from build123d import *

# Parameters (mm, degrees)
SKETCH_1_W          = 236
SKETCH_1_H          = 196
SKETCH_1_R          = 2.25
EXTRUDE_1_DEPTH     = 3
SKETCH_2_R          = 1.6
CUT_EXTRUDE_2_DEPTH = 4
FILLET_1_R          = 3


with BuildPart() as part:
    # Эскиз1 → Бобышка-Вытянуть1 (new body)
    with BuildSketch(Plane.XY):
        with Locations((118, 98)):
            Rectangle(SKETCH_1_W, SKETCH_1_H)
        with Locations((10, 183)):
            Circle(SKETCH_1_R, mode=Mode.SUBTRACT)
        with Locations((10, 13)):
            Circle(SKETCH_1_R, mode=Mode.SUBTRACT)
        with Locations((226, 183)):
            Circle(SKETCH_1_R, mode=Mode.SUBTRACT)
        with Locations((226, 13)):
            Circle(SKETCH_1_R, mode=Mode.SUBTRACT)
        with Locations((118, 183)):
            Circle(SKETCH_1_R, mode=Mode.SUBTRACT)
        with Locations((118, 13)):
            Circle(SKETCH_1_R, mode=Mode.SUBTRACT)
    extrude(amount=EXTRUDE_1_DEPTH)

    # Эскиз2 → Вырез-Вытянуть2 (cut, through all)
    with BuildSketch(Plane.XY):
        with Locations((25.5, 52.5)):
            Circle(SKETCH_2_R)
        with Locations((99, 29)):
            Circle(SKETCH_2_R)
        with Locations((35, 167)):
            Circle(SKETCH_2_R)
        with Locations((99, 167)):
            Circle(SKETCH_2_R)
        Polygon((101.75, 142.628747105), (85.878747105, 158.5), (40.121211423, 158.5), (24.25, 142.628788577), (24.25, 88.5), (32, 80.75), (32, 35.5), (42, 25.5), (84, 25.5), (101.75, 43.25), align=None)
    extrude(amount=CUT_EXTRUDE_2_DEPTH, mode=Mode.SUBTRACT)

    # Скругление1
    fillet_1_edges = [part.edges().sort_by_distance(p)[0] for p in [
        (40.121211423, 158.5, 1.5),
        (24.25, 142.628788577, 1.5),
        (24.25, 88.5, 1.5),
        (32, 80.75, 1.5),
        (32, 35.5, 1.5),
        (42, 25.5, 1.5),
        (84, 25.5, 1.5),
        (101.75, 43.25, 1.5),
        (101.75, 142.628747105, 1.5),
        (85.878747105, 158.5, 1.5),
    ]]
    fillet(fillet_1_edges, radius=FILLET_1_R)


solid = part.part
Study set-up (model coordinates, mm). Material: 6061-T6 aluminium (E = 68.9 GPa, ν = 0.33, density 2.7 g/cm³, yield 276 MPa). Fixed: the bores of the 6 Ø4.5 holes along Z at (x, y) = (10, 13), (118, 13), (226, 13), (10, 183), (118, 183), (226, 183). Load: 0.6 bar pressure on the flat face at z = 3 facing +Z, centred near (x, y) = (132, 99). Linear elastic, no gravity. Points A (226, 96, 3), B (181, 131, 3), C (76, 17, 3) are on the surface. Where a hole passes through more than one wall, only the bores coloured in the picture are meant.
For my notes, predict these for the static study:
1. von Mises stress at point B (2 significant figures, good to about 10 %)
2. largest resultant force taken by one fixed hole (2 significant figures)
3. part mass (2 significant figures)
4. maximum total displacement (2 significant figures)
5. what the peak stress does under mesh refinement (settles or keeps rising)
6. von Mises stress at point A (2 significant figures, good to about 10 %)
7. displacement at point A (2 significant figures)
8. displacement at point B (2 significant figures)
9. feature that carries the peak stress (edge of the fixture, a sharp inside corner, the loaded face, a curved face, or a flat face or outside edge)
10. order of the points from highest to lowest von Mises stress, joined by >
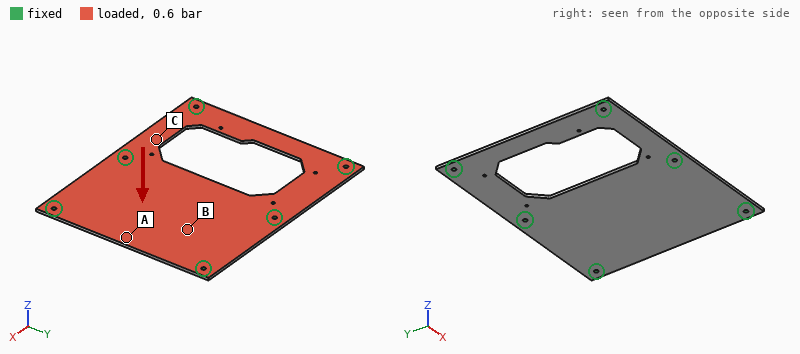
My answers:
35 MPa
520 N
300 g
1.2 mm
keeps rising
60 MPa
1.2 mm
0.99 mm
edge of the fixture
A > B > C
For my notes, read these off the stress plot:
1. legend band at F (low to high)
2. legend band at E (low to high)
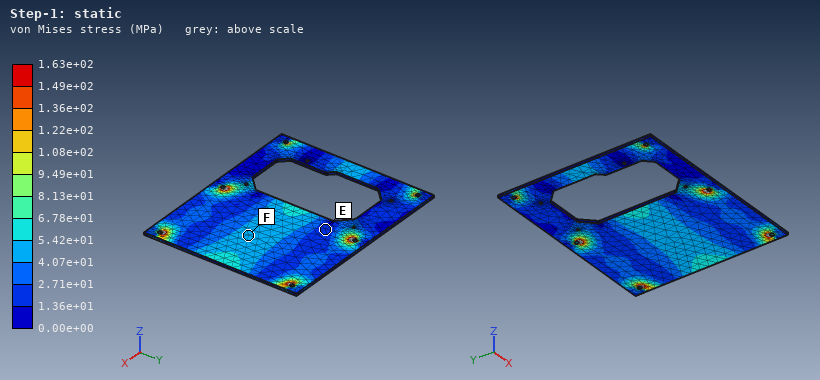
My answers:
4.07e+01 to 5.42e+01 MPa
1.36e+01 to 2.71e+01 MPa
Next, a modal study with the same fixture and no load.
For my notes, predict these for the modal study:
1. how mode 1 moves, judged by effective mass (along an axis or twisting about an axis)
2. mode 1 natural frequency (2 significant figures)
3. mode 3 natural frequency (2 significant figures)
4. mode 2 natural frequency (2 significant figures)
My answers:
along Z
450 Hz
720 Hz
580 Hz
